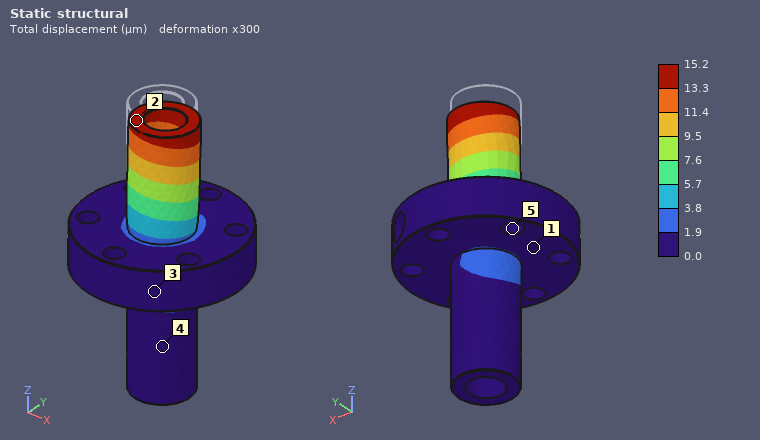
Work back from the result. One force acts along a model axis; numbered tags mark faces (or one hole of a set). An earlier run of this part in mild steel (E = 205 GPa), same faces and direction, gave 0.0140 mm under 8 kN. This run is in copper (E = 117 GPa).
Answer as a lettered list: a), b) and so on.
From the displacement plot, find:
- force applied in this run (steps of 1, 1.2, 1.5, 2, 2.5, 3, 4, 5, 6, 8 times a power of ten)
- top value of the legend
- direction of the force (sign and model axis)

a) 5 kN
b) 15.2 µm
c) -Z
